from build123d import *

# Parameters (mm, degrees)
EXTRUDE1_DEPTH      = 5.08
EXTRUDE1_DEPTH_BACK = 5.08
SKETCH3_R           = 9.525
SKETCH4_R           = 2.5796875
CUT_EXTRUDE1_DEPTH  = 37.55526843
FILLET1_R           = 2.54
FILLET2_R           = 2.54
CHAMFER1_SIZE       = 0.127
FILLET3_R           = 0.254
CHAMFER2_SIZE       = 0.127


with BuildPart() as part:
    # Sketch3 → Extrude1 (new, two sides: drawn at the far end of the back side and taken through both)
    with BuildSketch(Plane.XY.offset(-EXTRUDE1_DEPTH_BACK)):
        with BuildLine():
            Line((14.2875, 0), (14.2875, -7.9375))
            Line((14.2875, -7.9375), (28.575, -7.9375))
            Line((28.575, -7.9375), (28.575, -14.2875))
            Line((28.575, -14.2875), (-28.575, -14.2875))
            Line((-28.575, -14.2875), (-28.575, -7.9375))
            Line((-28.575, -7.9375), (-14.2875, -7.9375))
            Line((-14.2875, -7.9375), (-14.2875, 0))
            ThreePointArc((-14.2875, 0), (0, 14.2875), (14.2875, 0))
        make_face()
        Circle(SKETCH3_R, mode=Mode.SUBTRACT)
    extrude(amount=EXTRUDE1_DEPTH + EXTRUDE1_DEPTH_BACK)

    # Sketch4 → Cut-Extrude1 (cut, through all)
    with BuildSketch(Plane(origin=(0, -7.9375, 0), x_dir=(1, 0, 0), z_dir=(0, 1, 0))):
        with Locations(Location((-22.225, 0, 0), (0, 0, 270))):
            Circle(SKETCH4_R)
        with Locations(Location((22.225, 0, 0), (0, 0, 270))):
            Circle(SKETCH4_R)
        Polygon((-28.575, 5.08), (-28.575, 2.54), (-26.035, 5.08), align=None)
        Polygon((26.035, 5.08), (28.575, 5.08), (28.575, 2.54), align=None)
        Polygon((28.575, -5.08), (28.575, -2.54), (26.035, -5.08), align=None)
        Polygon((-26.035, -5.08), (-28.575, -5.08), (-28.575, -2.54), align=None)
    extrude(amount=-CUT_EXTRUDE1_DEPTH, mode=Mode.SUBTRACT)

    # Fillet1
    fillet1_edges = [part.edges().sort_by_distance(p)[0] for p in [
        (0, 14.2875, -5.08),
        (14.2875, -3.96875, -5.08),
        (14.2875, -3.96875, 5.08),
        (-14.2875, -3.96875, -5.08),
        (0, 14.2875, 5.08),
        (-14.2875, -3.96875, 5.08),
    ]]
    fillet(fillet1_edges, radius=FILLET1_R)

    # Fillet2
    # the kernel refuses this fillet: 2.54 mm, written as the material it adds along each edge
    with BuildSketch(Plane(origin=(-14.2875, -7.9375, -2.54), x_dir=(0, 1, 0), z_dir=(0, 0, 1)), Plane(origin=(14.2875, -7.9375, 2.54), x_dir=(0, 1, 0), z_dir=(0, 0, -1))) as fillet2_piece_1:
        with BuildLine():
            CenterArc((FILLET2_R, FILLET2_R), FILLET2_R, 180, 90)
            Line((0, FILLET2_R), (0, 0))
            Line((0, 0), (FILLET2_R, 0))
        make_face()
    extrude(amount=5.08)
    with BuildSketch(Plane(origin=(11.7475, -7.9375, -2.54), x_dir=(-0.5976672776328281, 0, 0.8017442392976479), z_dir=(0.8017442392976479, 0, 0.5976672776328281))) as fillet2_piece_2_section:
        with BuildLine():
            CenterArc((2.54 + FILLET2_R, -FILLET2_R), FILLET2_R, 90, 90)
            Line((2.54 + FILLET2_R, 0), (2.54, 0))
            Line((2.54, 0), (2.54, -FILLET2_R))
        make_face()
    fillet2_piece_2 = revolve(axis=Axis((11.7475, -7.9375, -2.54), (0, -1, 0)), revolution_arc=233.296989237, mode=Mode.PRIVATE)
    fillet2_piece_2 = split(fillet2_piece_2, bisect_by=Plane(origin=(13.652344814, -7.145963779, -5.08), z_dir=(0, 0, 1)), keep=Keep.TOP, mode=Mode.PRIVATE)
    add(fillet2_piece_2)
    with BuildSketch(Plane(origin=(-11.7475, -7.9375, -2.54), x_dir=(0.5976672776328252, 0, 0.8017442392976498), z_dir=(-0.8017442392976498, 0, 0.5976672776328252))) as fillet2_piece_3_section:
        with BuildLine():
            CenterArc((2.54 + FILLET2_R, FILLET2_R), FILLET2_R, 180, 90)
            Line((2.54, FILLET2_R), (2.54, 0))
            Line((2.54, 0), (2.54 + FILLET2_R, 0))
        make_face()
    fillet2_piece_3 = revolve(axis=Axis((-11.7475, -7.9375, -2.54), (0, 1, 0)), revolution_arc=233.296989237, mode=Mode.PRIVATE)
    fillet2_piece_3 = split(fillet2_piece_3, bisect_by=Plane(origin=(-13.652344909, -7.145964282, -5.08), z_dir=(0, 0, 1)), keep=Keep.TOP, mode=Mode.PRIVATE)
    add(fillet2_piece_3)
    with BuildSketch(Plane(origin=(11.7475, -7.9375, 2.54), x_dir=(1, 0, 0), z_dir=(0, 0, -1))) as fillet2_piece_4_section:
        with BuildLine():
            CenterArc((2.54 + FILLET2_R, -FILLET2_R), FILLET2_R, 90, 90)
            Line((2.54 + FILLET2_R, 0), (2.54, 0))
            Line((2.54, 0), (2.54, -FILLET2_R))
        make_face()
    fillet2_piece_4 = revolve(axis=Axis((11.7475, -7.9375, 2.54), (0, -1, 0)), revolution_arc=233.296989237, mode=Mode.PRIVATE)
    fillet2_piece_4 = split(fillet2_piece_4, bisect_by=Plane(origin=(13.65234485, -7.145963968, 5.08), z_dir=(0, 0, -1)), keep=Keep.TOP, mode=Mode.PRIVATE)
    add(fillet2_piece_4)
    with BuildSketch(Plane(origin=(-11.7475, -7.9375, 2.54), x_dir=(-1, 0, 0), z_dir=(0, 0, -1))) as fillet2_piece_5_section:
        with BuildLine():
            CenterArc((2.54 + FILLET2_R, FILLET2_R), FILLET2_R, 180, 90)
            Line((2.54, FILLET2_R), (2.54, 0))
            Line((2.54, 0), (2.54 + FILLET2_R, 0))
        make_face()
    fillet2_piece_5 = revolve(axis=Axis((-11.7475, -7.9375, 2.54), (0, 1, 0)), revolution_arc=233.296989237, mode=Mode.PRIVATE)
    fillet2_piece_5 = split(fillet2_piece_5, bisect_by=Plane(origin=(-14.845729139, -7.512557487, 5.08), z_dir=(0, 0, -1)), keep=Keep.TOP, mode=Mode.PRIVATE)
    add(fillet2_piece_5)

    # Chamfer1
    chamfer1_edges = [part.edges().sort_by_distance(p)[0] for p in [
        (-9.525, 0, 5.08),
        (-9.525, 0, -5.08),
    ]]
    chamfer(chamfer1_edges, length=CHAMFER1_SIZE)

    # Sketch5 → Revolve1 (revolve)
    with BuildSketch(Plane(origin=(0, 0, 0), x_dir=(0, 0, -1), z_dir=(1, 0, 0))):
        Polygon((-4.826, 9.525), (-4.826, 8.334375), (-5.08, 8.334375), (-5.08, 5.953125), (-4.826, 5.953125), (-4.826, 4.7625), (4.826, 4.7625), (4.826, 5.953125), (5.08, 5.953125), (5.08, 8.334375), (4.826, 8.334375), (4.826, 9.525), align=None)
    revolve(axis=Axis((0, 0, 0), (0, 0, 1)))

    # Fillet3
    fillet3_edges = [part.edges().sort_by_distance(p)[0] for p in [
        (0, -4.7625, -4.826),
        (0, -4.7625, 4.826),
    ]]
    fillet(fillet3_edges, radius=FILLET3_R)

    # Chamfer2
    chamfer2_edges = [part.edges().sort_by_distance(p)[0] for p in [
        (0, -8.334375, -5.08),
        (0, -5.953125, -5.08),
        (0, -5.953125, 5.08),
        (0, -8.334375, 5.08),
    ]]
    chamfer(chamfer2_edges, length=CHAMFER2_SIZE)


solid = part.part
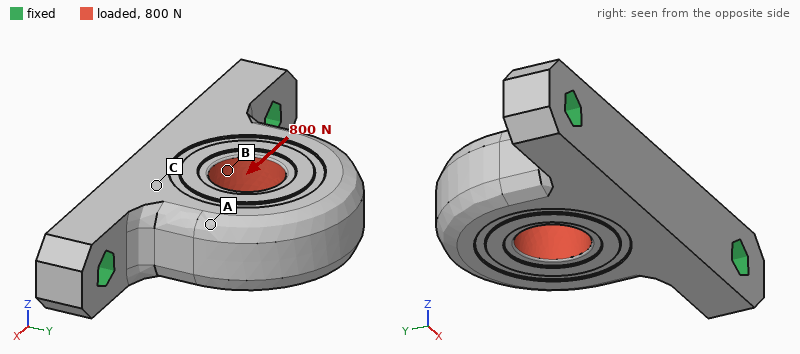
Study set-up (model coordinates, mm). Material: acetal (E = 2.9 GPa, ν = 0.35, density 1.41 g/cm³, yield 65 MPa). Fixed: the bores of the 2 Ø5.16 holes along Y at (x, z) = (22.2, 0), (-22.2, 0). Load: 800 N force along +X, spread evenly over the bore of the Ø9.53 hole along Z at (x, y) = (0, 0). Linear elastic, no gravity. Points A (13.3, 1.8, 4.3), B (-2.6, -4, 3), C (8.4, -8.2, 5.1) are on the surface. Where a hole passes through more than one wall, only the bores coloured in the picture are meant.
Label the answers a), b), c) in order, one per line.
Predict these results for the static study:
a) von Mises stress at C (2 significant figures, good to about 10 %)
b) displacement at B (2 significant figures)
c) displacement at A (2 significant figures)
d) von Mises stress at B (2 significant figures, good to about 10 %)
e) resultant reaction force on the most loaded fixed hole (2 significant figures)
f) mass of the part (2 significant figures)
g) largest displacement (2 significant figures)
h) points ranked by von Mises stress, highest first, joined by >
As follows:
a) 3.9 MPa
b) 0.048 mm
c) 0.090 mm
d) 8.9 MPa
e) 470 N
f) 11 g
g) 0.12 mm
h) B > C > A
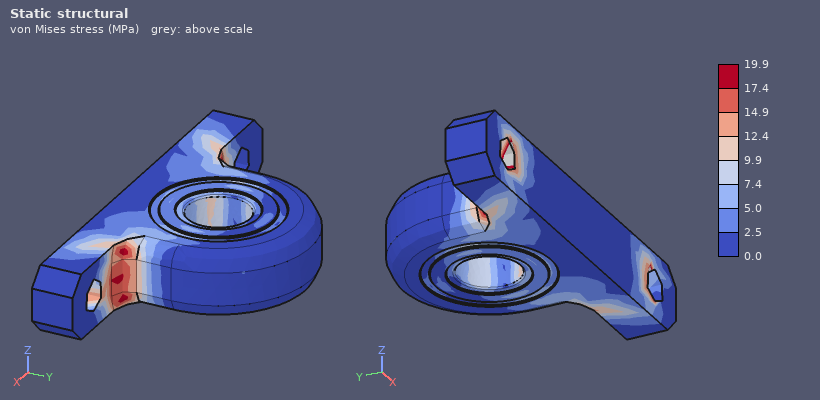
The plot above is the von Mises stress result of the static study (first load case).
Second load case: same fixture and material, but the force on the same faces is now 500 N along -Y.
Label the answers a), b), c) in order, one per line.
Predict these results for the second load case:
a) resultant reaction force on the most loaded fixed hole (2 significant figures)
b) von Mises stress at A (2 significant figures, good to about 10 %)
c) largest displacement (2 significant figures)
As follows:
a) 280 N
b) 2.4 MPa
c) 81 µm
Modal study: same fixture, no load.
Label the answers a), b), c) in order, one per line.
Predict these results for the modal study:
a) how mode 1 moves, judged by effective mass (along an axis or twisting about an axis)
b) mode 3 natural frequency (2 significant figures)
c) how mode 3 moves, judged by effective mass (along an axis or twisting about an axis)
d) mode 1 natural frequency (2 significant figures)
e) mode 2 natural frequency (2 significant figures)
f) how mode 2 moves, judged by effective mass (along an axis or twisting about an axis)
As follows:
a) along Z
b) 5000 Hz
c) along X
d) 1500 Hz
e) 4600 Hz
f) along Y
